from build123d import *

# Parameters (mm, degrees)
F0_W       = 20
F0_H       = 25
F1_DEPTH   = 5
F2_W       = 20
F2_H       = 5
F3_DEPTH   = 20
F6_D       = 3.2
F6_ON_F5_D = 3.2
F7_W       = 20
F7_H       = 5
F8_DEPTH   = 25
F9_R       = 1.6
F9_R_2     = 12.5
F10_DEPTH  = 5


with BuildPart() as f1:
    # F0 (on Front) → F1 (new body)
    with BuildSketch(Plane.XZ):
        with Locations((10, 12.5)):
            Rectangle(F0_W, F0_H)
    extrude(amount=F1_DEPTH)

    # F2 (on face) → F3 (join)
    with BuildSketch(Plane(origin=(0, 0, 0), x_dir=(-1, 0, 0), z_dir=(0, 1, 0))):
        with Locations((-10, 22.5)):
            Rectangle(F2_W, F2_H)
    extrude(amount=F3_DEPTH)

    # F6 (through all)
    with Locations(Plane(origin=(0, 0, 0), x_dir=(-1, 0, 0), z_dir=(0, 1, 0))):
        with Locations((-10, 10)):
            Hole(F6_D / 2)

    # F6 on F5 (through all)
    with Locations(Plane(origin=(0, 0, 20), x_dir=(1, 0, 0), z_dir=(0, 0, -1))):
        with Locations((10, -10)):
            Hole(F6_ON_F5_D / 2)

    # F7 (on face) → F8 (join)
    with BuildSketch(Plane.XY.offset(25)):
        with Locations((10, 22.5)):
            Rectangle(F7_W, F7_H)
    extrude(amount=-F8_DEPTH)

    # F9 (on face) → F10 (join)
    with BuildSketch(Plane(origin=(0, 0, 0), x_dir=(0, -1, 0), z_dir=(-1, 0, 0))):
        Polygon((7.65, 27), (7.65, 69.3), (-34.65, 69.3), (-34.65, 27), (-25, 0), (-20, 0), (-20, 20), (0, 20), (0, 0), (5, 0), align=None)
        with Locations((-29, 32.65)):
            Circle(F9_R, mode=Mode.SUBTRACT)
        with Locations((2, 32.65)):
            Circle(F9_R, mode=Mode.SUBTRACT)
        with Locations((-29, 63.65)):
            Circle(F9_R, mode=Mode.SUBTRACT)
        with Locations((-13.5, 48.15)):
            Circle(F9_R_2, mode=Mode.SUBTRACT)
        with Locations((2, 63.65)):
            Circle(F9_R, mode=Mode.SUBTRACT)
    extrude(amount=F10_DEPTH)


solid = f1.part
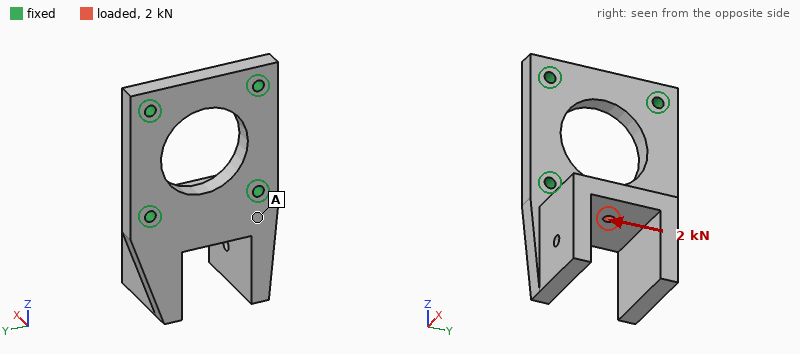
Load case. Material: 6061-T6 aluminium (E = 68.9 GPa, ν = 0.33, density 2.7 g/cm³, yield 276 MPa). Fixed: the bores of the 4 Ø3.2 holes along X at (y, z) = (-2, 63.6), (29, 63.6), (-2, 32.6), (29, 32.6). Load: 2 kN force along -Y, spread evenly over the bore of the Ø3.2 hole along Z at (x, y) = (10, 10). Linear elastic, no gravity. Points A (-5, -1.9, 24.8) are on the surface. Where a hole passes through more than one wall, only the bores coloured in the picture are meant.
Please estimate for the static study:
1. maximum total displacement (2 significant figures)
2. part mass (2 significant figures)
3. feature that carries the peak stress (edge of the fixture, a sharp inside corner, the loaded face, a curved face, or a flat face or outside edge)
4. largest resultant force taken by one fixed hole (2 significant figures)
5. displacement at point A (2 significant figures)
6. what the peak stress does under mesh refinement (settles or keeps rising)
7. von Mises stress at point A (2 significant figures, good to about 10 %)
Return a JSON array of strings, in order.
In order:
["58 µm", "44 g", "edge of the fixture", "1.4 kN", "13 µm", "keeps rising", "17 MPa"]
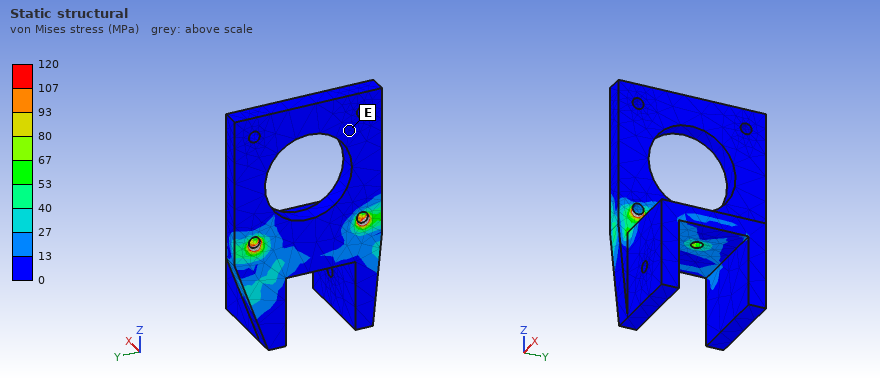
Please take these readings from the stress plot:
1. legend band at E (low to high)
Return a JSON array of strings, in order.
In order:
["0 to 13 MPa"]
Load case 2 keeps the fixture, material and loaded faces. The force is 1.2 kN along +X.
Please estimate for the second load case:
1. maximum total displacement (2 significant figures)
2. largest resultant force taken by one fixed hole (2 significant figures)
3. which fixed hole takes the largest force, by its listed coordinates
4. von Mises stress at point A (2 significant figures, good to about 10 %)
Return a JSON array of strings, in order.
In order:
["0.12 mm", "750 N", "(-2, 32.6)", "21 MPa"]
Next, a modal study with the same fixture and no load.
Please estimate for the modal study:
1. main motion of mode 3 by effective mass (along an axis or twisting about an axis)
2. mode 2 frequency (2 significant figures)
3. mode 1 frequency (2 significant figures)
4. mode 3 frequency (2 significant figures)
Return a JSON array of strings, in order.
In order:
["along Y", "4800 Hz", "2500 Hz", "6400 Hz"]
